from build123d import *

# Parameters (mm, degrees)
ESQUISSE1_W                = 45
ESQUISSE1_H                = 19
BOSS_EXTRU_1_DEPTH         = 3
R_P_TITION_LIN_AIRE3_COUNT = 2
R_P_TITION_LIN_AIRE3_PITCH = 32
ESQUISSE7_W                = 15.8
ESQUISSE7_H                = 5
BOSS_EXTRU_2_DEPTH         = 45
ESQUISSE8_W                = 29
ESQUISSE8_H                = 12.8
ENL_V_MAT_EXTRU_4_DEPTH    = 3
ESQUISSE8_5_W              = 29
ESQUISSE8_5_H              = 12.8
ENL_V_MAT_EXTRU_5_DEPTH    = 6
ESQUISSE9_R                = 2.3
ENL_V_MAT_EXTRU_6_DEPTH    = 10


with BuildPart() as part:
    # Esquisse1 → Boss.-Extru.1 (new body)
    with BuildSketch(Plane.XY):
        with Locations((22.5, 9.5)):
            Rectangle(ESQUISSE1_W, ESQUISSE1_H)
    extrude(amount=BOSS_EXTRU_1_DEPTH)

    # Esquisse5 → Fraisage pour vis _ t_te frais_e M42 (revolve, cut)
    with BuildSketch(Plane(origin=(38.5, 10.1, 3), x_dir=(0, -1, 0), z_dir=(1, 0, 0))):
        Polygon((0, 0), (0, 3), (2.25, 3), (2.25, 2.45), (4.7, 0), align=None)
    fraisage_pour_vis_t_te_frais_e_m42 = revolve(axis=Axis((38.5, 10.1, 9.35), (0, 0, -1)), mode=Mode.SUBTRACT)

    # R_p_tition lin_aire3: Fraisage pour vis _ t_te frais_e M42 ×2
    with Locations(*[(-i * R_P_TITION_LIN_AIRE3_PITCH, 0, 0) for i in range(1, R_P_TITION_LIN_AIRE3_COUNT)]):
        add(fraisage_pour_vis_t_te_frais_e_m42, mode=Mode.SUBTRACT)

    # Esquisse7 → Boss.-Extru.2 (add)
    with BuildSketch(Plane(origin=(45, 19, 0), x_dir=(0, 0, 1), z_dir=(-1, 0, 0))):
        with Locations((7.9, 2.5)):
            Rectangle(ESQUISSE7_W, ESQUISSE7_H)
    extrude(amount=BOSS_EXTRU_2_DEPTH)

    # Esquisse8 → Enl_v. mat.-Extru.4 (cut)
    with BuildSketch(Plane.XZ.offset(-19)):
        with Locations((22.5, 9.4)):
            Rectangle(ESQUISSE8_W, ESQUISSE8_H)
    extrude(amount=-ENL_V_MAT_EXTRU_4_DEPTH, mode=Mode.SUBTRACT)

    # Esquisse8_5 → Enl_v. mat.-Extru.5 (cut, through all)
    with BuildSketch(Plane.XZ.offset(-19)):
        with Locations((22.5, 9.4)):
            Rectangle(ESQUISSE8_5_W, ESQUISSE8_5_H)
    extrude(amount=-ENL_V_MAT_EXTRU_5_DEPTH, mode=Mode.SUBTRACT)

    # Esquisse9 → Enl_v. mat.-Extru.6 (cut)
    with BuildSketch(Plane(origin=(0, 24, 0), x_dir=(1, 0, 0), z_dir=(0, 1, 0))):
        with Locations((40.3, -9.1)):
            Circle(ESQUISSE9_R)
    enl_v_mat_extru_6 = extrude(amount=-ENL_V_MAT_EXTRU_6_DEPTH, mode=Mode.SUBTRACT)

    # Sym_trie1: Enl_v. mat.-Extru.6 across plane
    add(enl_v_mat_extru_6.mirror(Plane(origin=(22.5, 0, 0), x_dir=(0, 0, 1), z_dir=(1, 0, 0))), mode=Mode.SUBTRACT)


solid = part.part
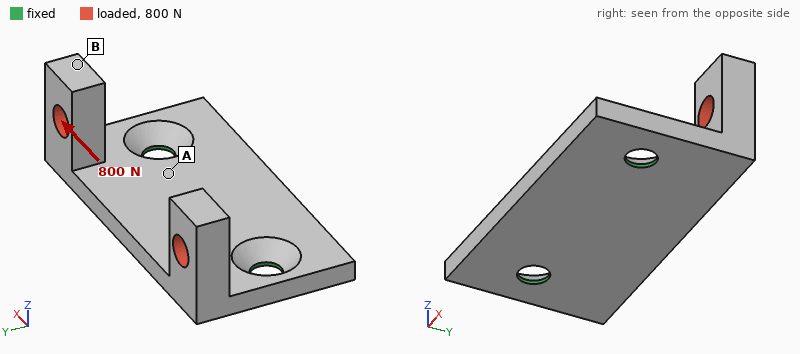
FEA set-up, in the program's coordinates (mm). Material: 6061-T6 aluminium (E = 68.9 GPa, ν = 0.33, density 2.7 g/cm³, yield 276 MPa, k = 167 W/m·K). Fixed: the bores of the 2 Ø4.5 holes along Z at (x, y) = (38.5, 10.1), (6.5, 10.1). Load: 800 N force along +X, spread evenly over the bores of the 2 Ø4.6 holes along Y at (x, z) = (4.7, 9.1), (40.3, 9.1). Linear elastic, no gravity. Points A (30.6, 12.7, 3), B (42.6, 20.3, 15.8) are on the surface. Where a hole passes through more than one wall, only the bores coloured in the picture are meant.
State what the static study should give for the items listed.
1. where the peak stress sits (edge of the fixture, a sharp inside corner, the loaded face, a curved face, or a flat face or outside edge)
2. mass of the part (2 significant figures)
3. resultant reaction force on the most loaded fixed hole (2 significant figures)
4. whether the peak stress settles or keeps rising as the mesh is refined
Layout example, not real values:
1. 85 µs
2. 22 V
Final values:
1. edge of the fixture
2. 10 g
3. 510 N
4. keeps rising
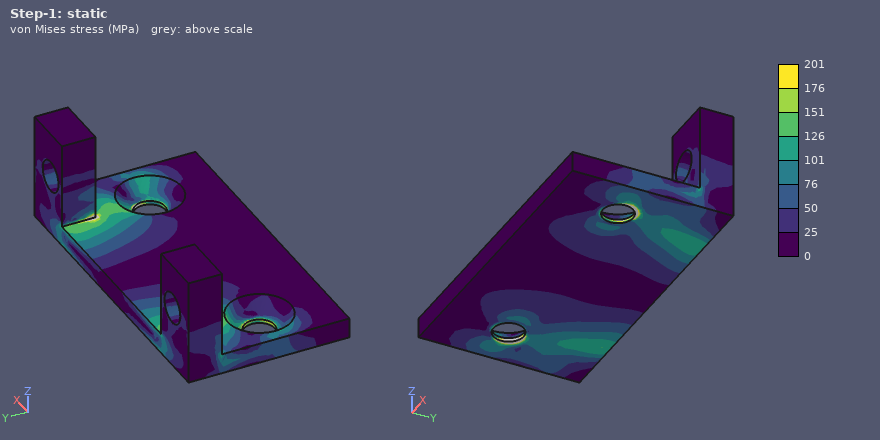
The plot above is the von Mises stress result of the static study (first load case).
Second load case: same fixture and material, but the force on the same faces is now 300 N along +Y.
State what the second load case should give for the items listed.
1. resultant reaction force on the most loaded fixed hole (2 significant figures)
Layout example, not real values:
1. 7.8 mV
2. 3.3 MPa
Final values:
1. 160 N
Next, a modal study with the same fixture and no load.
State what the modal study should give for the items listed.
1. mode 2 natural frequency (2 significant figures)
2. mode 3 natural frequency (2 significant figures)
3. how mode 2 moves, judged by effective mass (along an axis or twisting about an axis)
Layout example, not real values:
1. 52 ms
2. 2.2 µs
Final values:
1. 4700 Hz
2. 6600 Hz
3. twisting about Y
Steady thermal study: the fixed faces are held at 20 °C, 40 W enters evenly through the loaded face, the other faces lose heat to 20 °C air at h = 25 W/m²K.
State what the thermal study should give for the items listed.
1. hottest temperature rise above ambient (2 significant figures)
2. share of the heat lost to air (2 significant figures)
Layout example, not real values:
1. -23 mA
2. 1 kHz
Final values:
1. 69 K
2. 5.1 %
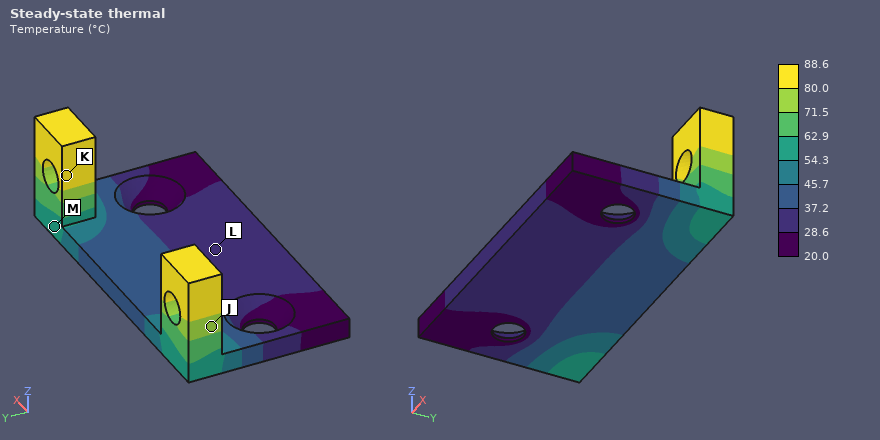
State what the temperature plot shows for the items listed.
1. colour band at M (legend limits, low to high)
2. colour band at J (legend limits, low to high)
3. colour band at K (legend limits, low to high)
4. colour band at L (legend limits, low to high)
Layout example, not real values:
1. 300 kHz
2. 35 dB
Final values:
1. 54.3 to 62.9 °C
2. 71.5 to 80.0 °C
3. 80.0 to 88.6 °C
4. 28.6 to 37.2 °C
